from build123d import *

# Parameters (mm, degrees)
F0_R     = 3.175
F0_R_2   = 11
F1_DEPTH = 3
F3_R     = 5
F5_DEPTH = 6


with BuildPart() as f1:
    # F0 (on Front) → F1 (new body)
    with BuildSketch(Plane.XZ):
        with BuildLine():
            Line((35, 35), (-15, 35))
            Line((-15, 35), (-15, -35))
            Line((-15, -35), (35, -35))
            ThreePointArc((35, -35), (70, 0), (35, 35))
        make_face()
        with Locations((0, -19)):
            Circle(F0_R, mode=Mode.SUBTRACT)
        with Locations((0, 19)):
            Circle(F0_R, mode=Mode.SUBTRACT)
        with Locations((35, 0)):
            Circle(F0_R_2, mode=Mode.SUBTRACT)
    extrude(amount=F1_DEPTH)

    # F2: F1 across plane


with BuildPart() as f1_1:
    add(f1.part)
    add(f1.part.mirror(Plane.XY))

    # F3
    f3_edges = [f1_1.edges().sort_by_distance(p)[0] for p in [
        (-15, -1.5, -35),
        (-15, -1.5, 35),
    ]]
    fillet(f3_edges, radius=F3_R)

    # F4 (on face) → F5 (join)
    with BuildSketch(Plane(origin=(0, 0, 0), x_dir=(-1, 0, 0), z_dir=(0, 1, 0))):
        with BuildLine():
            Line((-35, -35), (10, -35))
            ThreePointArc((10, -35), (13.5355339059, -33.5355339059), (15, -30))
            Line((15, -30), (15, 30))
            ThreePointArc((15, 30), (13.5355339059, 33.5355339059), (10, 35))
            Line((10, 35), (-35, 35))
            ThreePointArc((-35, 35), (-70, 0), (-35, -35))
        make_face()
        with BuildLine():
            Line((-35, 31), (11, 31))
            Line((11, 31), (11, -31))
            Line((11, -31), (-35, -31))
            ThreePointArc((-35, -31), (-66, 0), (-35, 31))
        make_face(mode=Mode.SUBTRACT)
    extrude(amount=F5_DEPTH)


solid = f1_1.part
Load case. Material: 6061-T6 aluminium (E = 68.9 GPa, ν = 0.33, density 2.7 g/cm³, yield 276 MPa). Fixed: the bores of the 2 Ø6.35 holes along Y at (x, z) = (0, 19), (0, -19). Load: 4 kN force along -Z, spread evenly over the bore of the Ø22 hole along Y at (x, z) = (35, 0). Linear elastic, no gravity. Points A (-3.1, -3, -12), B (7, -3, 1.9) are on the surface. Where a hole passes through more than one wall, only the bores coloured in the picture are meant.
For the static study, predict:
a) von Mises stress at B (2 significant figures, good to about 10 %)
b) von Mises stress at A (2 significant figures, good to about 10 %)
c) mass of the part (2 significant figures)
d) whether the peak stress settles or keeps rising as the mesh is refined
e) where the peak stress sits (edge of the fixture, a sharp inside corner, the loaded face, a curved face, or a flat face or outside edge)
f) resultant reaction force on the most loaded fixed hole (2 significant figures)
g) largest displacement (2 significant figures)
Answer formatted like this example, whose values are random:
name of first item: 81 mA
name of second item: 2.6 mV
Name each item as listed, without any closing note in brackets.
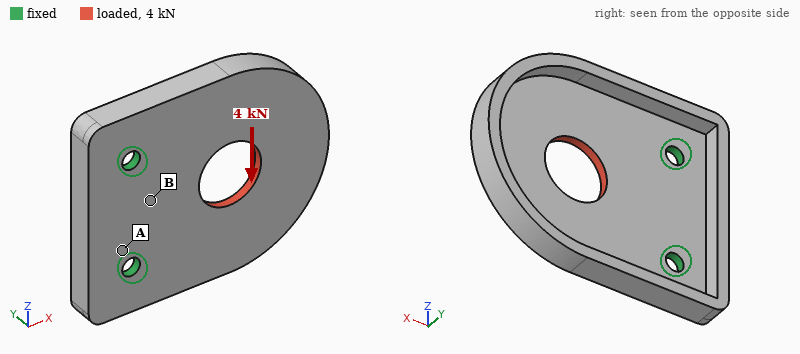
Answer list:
von Mises stress at B: 52 MPa
von Mises stress at A: 18 MPa
mass of the part: 57 g
whether the peak stress settles or keeps rising as the mesh is refined: keeps rising
where the peak stress sits: edge of the fixture
resultant reaction force on the most loaded fixed hole: 3.8 kN
largest displacement: 0.10 mm
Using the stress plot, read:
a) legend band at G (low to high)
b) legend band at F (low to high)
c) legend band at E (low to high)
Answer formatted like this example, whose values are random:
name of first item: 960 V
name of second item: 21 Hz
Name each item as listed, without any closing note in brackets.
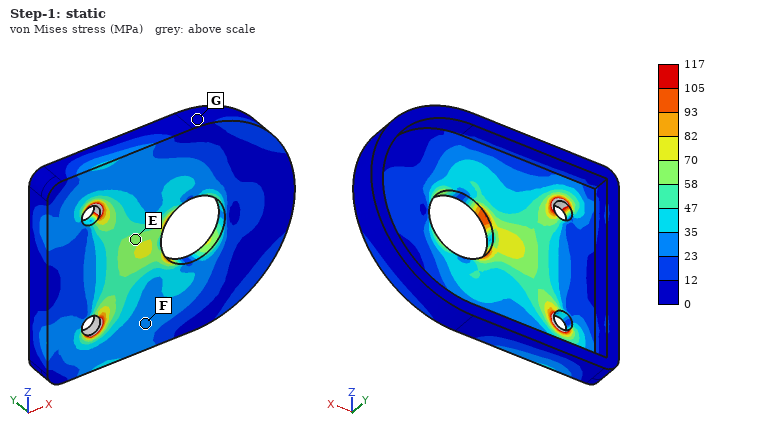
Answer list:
legend band at G: 0 to 12 MPa
legend band at F: 23 to 35 MPa
legend band at E: 58 to 70 MPa
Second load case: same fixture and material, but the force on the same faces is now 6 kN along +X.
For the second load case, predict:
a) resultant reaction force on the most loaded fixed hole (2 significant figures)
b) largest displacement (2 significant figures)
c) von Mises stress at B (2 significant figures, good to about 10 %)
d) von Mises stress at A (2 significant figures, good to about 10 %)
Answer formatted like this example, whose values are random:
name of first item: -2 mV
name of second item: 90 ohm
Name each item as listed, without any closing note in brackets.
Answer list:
resultant reaction force on the most loaded fixed hole: 3.0 kN
largest displacement: 57 µm
von Mises stress at B: 17 MPa
von Mises stress at A: 21 MPa
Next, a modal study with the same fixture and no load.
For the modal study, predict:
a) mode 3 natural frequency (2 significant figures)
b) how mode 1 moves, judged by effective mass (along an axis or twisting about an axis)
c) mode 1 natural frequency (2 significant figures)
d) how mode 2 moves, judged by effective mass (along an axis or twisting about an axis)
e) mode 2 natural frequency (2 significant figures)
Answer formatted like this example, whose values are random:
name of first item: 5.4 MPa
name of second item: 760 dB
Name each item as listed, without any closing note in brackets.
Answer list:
mode 3 natural frequency: 4400 Hz
how mode 1 moves, judged by effective mass: along Y
mode 1 natural frequency: 800 Hz
how mode 2 moves, judged by effective mass: twisting about X
mode 2 natural frequency: 1800 Hz
